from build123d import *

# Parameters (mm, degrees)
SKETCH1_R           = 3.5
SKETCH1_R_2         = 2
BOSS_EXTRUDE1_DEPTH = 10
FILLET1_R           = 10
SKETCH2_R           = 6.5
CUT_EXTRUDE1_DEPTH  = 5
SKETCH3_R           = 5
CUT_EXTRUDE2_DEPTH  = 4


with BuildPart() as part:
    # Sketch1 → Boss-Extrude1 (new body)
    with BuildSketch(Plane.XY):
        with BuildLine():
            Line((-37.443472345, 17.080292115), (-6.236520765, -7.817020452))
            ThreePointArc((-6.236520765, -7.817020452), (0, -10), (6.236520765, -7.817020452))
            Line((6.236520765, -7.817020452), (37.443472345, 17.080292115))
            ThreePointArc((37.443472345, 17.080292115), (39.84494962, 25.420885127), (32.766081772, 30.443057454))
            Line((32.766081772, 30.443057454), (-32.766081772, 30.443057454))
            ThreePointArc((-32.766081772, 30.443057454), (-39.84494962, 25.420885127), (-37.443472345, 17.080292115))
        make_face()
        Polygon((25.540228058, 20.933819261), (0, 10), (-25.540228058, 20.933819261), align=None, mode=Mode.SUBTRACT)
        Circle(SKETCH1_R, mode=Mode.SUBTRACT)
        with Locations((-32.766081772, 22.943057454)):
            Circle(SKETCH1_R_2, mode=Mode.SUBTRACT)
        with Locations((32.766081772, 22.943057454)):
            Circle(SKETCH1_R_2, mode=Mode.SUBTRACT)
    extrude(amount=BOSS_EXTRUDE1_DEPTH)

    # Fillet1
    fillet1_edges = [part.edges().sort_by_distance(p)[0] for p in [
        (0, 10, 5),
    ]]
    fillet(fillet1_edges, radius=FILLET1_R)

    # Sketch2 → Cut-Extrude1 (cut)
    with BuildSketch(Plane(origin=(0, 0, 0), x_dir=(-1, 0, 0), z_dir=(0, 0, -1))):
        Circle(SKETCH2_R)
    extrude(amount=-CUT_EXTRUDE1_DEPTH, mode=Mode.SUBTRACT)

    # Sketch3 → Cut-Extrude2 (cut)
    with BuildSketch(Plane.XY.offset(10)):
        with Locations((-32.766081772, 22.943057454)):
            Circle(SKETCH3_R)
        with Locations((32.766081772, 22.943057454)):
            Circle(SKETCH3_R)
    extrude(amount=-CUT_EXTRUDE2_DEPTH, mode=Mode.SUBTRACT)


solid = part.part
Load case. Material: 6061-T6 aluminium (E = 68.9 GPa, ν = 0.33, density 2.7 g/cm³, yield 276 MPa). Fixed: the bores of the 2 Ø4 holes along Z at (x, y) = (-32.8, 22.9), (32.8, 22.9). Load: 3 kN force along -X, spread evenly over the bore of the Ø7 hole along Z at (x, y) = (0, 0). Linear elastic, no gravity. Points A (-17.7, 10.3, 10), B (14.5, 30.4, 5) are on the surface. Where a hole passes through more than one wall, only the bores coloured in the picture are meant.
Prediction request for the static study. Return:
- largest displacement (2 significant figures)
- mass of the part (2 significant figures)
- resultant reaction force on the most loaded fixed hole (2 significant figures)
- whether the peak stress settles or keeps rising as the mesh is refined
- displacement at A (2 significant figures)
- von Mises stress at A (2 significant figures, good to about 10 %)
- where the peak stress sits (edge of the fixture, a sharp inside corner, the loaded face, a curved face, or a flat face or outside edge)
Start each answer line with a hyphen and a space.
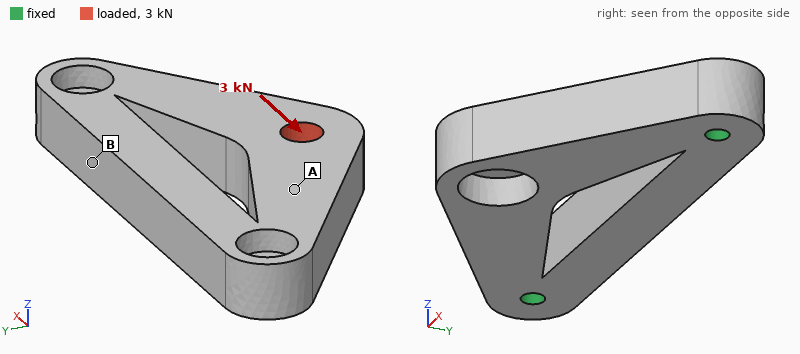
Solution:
- 17 µm
- 46 g
- 1.8 kN
- keeps rising
- 8.6 µm
- 15 MPa
- edge of the fixture
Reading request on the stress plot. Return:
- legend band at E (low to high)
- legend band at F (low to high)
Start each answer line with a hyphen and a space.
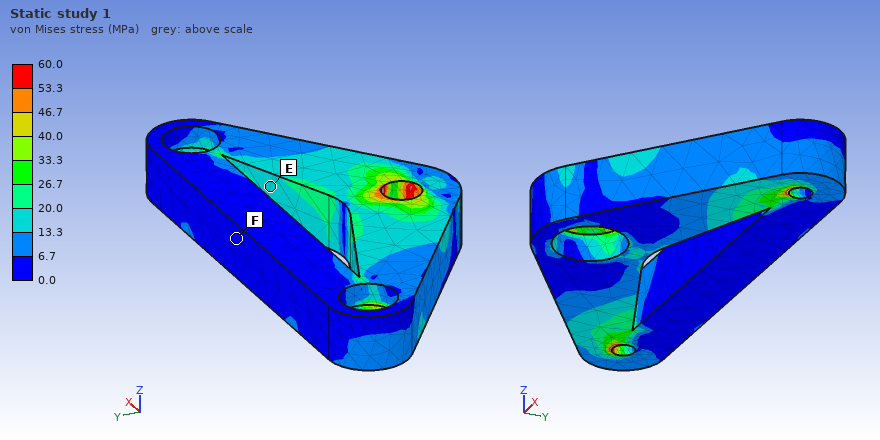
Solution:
- 13.3 to 20.0 MPa
- 0.0 to 6.7 MPa
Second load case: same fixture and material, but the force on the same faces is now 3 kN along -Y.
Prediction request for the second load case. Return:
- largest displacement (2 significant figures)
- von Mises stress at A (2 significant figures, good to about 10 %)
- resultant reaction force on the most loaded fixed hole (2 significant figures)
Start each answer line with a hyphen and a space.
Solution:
- 0.11 mm
- 36 MPa
- 2.0 kN
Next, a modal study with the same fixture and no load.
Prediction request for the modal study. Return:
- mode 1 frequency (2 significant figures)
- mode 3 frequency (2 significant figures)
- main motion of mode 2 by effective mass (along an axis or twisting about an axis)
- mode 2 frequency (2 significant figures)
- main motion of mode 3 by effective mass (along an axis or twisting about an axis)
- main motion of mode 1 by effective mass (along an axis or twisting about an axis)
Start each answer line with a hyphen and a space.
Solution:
- 4000 Hz
- 10 kHz
- along Z
- 9000 Hz
- along Y
- along Z
